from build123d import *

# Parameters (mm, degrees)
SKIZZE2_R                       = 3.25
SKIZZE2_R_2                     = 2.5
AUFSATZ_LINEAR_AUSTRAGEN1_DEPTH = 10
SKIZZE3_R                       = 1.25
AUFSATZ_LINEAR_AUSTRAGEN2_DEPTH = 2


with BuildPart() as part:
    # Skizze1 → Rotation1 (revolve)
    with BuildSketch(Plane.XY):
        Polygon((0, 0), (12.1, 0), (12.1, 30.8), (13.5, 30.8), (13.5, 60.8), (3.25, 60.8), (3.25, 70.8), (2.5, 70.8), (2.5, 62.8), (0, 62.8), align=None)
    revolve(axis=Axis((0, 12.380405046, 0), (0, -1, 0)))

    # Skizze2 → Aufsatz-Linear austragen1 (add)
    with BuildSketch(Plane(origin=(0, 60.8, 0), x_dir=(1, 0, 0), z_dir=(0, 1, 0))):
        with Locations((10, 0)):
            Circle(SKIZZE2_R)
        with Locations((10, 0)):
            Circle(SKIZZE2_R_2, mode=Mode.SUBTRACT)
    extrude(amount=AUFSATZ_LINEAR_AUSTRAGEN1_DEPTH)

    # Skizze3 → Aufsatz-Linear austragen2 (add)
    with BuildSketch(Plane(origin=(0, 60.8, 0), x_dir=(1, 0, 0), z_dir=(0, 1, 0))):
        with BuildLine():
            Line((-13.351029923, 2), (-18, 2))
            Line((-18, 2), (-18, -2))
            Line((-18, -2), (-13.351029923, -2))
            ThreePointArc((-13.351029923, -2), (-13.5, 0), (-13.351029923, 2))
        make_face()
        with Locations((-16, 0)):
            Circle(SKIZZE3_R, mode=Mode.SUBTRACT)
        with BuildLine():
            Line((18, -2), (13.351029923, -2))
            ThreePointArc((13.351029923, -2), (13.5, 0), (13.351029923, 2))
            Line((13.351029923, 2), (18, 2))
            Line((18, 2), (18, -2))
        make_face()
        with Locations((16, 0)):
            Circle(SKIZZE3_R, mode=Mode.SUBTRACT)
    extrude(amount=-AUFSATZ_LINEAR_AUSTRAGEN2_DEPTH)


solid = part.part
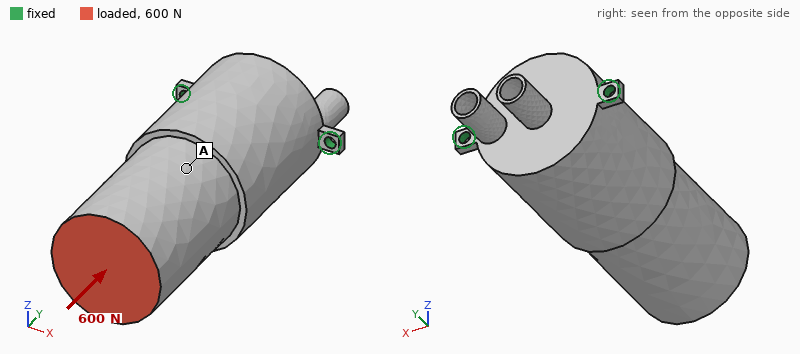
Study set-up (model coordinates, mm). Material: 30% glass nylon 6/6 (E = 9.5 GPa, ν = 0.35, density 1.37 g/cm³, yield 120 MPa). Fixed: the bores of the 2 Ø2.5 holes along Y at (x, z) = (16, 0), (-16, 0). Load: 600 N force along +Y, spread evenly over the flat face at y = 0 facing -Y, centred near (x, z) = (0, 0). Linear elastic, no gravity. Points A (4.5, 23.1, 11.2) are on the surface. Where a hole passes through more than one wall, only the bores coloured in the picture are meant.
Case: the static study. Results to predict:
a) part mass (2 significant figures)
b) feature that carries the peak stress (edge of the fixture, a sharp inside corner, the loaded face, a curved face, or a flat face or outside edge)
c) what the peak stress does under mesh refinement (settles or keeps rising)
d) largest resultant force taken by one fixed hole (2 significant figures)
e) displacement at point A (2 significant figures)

43 g
edge of the fixture
keeps rising
330 N
52 µm
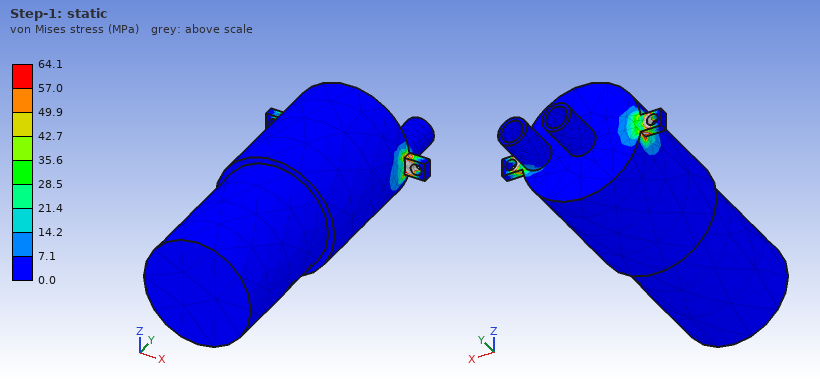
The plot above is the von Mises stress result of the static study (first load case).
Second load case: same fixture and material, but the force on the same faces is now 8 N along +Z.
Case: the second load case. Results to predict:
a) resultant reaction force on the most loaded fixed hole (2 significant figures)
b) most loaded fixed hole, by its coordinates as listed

4.3 N
(-16, 0)
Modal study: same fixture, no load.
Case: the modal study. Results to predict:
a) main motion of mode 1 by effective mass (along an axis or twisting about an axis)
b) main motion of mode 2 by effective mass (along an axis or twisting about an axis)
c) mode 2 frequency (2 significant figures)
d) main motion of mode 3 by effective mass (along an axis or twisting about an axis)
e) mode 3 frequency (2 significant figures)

along Z
along X
1100 Hz
along Y
2600 Hz
